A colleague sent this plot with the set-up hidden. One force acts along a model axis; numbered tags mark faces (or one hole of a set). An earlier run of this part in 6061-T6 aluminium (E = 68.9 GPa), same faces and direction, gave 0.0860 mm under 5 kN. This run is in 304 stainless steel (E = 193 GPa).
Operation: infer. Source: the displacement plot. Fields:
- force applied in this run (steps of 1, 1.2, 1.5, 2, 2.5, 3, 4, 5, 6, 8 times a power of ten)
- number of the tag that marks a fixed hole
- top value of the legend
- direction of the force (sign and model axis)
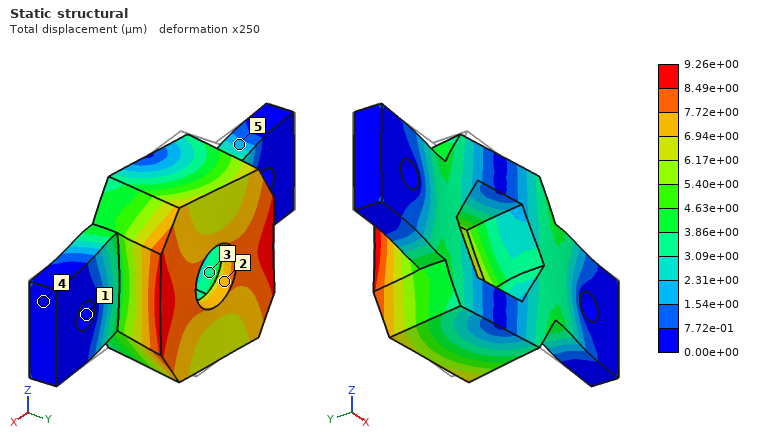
1.5 kN
1
9.26e+00 µm
+X
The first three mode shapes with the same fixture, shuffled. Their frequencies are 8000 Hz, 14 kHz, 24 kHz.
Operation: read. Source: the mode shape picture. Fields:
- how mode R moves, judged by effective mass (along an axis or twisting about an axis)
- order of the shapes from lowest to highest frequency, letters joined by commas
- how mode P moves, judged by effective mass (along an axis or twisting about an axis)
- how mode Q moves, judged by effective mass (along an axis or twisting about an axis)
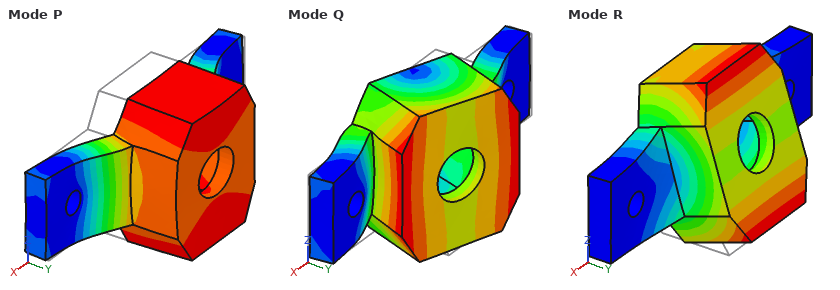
along Z
R, P, Q
along Y
along X
